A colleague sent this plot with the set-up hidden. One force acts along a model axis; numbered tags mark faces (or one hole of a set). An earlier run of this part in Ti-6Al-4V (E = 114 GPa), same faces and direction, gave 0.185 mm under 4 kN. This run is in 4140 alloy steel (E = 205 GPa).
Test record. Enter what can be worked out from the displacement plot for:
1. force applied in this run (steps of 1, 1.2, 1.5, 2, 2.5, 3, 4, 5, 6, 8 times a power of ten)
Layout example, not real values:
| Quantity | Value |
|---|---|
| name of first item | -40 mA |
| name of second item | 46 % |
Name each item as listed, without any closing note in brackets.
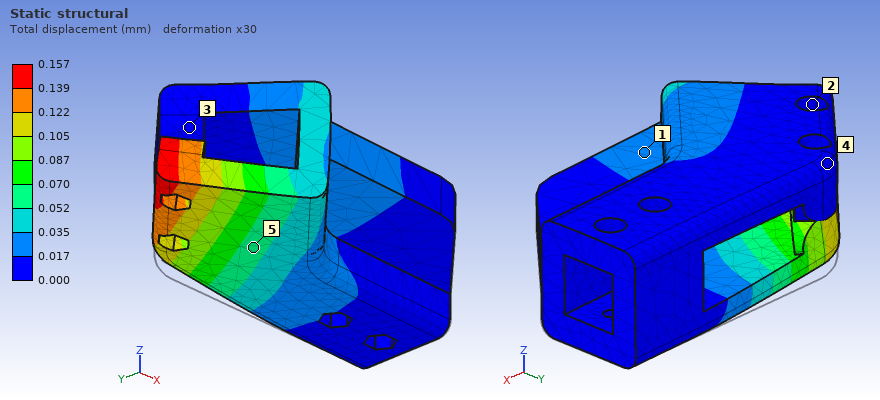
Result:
| Quantity | Value |
|---|---|
| force applied in this run | 6 kN |
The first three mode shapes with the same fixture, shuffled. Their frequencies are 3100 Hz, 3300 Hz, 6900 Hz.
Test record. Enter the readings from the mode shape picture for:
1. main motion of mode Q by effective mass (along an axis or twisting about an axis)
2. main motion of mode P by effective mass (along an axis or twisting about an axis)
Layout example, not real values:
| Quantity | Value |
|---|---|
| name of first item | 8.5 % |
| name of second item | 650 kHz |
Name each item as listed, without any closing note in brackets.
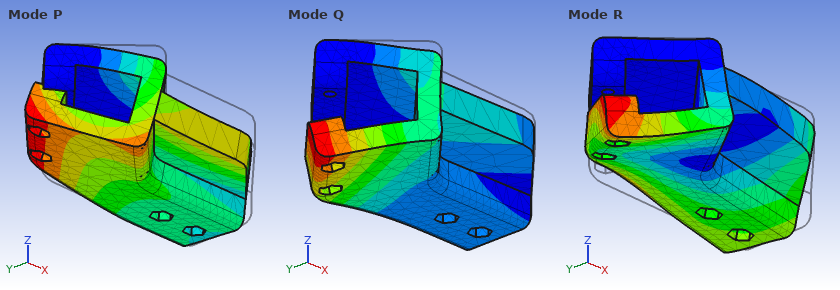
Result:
| Quantity | Value |
|---|---|
| main motion of mode Q by effective mass | along Z |
| main motion of mode P by effective mass | along Y |
